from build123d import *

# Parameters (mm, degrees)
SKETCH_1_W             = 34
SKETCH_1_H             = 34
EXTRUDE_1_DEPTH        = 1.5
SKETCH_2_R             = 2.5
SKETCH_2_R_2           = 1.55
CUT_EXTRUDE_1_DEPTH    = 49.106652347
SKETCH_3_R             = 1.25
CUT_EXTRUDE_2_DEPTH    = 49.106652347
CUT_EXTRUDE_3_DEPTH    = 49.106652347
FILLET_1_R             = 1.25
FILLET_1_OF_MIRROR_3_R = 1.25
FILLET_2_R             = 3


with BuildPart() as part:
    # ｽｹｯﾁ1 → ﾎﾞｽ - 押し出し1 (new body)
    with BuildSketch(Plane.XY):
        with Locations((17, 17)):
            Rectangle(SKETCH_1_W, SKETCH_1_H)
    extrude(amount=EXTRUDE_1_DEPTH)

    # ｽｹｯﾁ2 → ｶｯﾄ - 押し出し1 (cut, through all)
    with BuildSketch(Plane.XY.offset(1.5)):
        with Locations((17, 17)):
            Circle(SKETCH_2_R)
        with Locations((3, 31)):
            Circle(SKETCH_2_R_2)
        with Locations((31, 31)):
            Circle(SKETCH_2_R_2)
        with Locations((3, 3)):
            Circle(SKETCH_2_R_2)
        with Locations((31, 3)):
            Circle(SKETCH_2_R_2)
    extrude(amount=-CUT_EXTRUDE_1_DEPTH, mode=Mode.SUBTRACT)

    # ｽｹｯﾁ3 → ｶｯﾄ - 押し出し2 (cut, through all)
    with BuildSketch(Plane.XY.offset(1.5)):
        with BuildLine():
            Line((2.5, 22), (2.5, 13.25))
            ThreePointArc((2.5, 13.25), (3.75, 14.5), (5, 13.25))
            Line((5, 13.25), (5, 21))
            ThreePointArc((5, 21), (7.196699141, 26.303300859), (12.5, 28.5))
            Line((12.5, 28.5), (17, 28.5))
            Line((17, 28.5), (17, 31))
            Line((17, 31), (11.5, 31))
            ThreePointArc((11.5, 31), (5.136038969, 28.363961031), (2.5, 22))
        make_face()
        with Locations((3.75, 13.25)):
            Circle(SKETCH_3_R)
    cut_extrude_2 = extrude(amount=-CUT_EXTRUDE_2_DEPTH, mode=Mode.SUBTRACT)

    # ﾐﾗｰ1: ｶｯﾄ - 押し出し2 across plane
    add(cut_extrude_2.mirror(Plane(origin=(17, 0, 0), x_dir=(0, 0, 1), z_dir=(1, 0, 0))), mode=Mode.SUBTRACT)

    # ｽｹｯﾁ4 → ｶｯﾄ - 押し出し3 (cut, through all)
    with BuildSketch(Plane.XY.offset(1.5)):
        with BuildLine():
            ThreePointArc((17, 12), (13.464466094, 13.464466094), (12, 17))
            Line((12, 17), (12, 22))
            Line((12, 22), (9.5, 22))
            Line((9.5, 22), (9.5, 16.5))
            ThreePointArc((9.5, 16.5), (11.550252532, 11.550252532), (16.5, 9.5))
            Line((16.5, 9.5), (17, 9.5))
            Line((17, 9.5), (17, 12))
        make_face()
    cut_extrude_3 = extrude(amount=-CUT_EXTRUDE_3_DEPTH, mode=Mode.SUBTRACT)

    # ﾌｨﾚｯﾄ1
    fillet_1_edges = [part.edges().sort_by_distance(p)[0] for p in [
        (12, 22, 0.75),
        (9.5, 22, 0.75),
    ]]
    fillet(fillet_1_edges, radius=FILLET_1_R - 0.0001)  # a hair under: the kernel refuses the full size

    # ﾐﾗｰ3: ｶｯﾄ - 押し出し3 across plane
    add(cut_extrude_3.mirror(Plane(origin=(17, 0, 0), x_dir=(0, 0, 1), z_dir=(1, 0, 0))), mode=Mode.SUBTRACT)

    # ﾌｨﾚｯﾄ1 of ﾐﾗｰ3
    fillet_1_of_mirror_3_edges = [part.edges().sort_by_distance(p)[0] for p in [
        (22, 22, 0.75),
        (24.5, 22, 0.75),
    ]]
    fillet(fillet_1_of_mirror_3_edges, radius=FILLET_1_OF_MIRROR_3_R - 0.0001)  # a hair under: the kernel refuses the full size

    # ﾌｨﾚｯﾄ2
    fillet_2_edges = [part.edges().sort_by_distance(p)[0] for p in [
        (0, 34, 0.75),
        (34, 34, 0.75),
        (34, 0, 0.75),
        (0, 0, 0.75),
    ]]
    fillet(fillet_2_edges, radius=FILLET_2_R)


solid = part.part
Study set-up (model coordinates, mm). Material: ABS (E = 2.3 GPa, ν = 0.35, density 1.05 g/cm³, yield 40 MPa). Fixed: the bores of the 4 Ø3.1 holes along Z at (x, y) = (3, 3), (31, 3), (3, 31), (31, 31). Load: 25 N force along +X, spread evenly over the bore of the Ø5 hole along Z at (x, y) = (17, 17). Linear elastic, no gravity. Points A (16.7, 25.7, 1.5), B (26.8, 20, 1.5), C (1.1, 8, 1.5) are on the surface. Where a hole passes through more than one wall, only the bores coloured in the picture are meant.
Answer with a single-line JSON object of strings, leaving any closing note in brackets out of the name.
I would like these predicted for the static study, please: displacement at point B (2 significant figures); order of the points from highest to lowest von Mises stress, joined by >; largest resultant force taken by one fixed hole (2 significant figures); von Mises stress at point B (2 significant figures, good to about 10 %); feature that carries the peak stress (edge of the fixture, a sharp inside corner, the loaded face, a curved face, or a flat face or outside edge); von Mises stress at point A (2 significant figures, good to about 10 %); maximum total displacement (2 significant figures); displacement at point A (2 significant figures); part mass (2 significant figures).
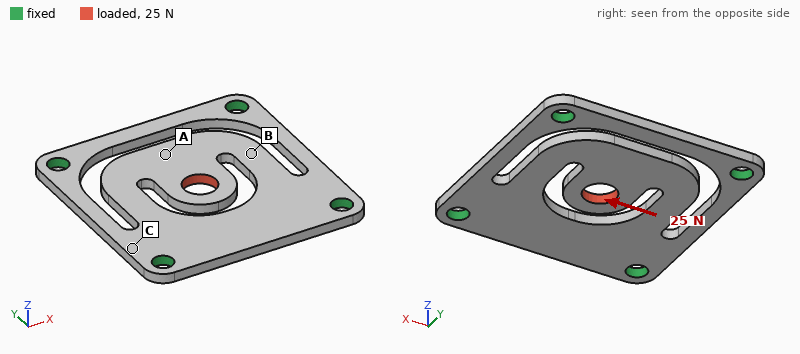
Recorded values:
{"displacement at point B": "0.096 mm", "order of the points from highest to lowest von Mises stress, joined by >": "B > A > C", "largest resultant force taken by one fixed hole": "15 N", "von Mises stress at point B": "4.8 MPa", "feature that carries the peak stress": "a curved face", "von Mises stress at point A": "3.2 MPa", "maximum total displacement": "0.22 mm", "displacement at point A": "0.13 mm", "part mass": "1.4 g"}
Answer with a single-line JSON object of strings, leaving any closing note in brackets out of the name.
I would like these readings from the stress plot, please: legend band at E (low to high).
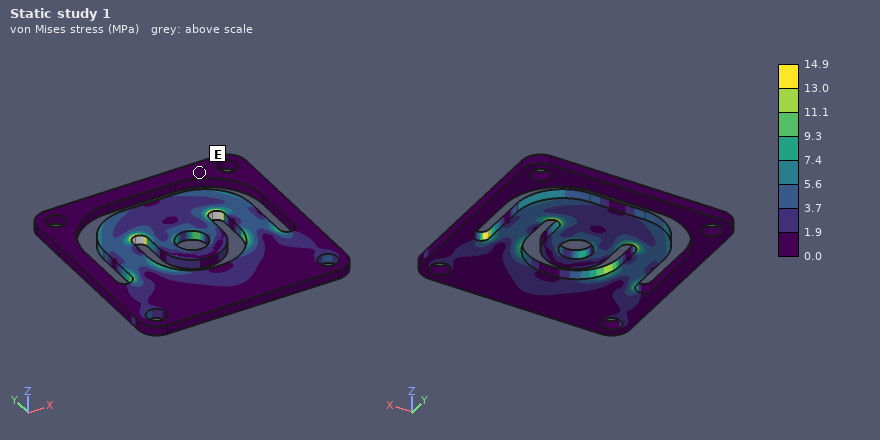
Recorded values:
{"legend band at E": "0.0 to 1.9 MPa"}
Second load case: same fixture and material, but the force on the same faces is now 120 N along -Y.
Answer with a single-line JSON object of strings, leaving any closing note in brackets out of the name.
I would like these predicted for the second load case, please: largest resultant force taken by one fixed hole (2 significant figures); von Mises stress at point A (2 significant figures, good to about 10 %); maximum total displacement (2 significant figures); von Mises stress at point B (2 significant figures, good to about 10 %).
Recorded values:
{"largest resultant force taken by one fixed hole": "61 N", "von Mises stress at point A": "5.8 MPa", "maximum total displacement": "0.20 mm", "von Mises stress at point B": "8.3 MPa"}
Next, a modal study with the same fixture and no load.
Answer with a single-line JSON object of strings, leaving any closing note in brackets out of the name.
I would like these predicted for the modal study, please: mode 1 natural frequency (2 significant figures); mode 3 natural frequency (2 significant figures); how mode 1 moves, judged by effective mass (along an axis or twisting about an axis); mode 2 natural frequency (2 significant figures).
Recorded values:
{"mode 1 natural frequency": "570 Hz", "mode 3 natural frequency": "1600 Hz", "how mode 1 moves, judged by effective mass": "along Z", "mode 2 natural frequency": "1500 Hz"}
